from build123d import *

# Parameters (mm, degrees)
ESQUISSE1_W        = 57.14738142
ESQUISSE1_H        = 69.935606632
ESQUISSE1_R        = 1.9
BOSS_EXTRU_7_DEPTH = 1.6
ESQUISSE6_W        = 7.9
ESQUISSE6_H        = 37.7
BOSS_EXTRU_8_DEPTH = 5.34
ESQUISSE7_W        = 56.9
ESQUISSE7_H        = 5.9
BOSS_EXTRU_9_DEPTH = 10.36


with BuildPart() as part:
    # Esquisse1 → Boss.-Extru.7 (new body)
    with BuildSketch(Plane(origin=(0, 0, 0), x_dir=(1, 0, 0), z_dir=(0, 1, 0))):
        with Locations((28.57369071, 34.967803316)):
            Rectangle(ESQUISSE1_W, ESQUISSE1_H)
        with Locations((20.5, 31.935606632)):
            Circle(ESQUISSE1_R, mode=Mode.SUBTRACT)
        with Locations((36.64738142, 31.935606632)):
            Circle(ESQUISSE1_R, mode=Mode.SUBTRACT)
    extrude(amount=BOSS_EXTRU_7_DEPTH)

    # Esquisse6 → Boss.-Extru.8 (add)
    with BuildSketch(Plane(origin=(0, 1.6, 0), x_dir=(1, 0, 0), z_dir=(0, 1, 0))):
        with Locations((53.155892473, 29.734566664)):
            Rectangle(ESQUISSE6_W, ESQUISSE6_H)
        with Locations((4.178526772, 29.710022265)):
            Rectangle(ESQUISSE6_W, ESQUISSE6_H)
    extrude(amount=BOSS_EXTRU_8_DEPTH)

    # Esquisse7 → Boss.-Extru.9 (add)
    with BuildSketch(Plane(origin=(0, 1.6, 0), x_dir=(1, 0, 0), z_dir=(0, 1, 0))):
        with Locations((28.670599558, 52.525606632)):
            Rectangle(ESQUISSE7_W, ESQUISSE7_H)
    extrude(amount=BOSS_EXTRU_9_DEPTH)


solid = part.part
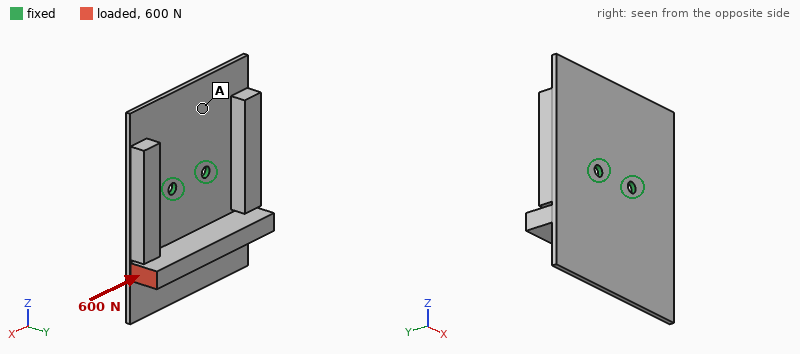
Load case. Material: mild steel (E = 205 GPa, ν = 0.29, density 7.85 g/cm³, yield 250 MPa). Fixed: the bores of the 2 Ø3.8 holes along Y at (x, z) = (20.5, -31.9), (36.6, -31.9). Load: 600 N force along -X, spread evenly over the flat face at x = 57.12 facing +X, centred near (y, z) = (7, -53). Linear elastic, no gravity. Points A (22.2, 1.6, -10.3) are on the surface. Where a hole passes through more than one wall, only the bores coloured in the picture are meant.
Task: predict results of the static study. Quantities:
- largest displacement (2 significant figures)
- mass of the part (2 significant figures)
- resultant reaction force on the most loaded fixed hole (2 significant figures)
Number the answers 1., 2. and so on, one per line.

1. 72 µm
2. 100 g
3. 730 N
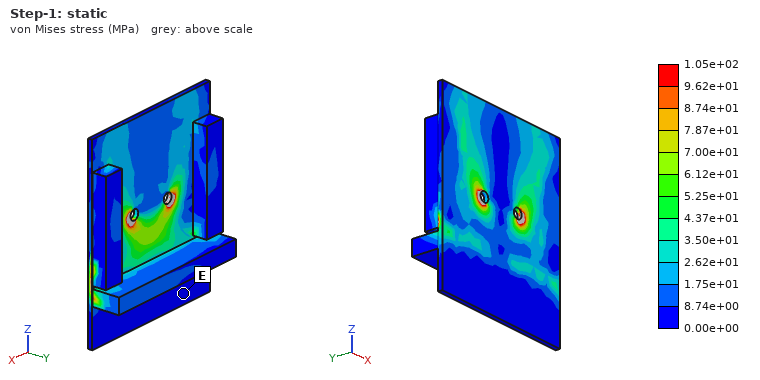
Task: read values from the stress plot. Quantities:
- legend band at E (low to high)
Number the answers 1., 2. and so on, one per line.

1. 0.00e+00 to 8.74e+00 MPa
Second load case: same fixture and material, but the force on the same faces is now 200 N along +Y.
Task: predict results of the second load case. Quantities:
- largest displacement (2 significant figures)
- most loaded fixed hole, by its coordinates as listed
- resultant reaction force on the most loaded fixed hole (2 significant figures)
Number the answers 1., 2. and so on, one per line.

1. 0.30 mm
2. (36.6, -31.9)
3. 320 N
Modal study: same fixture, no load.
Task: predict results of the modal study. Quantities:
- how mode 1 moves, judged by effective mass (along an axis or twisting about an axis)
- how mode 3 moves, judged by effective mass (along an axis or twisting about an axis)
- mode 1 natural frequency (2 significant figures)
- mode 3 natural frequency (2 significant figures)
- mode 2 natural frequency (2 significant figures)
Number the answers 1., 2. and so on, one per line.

1. along Y
2. along Y
3. 810 Hz
4. 2000 Hz
5. 1400 Hz
